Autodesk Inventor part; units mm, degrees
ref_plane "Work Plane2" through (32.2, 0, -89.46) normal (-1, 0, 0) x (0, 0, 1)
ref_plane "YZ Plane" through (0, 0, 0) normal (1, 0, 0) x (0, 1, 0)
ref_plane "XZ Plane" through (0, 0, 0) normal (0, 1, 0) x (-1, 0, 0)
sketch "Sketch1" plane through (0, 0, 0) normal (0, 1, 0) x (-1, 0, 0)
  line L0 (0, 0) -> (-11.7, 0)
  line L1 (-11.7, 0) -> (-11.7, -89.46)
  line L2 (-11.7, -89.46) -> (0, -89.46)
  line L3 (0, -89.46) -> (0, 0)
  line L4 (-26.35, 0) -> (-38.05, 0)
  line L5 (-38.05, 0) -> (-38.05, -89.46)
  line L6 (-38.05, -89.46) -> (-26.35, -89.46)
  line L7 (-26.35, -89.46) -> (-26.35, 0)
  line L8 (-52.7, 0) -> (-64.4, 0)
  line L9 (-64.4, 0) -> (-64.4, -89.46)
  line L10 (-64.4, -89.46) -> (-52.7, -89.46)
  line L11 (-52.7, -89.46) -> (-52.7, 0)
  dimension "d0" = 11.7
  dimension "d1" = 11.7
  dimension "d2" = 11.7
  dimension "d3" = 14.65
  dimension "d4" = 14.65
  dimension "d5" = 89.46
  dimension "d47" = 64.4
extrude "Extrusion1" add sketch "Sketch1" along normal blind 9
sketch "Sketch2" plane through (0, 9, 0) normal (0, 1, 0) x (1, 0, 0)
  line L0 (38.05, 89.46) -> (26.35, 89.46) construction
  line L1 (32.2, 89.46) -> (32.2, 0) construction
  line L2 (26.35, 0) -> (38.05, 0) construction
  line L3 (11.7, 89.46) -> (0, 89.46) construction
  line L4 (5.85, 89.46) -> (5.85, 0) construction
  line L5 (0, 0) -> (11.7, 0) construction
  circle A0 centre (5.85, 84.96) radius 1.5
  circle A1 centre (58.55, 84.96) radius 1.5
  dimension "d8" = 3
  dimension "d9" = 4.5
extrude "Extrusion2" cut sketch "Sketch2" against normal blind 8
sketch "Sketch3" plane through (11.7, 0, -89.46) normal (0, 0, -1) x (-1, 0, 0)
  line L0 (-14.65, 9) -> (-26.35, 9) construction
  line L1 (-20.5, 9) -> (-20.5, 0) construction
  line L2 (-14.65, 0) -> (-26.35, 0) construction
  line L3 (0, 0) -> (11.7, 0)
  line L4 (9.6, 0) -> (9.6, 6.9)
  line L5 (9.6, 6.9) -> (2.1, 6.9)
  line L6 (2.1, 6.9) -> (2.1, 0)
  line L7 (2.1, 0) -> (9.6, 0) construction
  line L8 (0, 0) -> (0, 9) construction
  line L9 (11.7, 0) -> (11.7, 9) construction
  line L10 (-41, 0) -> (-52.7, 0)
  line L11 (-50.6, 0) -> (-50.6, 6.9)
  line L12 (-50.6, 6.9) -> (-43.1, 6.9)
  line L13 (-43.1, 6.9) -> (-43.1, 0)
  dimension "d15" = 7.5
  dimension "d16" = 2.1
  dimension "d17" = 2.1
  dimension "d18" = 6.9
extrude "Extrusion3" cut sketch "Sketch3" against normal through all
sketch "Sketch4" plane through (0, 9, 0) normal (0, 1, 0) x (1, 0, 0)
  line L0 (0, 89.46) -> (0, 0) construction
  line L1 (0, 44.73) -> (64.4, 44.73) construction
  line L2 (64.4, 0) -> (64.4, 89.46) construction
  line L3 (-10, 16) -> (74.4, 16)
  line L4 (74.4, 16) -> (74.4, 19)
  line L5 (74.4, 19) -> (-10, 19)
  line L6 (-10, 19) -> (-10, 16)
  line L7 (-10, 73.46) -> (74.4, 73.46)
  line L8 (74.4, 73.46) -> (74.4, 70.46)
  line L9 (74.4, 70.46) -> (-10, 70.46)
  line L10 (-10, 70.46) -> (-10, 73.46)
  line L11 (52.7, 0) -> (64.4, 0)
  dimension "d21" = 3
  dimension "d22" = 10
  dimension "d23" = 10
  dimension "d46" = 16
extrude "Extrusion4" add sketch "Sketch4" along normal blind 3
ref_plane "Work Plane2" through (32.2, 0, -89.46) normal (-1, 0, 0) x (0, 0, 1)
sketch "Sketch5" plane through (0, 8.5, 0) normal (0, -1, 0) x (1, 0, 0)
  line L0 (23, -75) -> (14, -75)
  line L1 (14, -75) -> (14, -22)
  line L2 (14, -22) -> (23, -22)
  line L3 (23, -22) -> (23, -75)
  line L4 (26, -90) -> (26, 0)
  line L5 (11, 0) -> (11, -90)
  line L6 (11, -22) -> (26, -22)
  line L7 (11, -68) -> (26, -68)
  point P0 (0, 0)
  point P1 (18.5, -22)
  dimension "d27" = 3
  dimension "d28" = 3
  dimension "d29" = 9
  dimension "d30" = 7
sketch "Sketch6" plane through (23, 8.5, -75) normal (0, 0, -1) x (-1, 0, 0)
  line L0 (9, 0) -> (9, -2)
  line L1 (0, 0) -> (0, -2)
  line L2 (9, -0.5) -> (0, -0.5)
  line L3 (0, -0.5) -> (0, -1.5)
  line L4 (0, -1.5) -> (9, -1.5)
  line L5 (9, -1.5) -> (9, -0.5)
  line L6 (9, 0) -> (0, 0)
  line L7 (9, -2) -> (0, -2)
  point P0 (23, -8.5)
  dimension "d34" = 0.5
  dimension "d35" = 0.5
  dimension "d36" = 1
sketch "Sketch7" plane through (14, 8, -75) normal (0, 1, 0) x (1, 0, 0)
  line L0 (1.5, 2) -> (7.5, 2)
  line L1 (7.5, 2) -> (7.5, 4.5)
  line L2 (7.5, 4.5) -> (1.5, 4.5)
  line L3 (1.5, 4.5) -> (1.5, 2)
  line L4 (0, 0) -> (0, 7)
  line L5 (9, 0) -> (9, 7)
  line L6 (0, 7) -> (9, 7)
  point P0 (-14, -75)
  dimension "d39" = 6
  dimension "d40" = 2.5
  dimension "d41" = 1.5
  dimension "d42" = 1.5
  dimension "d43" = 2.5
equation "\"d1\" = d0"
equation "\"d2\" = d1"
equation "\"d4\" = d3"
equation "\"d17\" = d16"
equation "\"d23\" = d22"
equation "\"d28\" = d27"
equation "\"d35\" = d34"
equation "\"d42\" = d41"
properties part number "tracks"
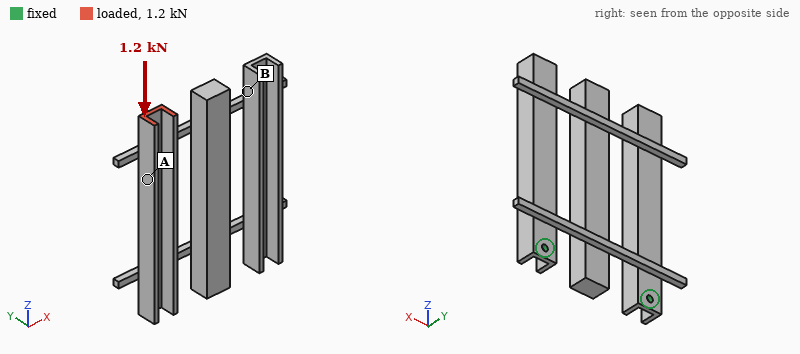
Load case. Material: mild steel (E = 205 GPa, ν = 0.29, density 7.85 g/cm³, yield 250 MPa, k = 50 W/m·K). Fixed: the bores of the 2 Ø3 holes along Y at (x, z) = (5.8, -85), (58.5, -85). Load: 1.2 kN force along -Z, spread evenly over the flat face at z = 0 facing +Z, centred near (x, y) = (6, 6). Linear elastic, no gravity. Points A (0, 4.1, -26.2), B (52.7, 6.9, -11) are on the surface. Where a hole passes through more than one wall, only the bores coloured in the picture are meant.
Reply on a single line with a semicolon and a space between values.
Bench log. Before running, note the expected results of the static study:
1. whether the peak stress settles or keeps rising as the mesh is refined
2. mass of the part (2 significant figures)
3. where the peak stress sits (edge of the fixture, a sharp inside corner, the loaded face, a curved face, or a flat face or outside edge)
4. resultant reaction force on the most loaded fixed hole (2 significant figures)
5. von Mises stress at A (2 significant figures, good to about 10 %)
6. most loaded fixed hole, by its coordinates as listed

keeps rising; 160 g; edge of the fixture; 1.2 kN; 23 MPa; (5.8, -85)
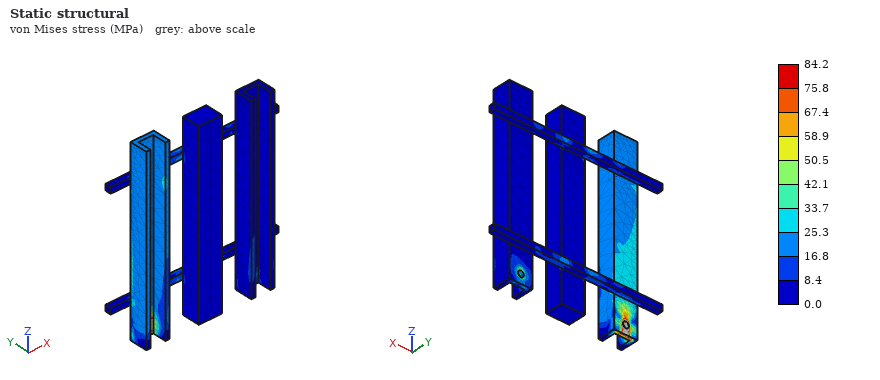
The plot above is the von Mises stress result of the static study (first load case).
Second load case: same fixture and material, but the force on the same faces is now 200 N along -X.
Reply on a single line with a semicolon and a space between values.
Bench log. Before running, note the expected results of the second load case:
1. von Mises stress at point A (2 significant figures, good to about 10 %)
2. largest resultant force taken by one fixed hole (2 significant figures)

31 MPa; 210 N
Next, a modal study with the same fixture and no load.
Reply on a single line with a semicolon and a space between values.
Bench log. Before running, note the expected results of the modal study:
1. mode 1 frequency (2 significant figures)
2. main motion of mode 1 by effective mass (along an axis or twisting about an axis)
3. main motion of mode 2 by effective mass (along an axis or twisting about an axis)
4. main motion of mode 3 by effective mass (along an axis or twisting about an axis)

380 Hz; along Y; along X; along X
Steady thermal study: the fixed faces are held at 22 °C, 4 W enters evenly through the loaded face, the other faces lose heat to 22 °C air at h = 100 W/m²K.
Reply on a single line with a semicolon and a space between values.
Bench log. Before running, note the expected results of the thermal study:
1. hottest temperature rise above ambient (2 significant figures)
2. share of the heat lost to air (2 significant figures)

31 K; 97 %
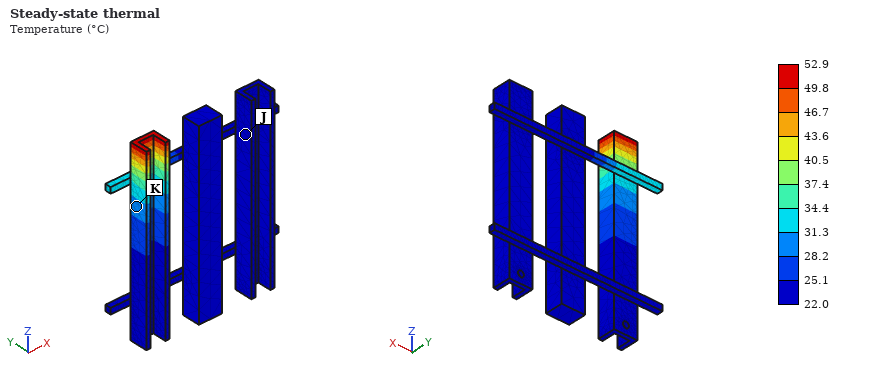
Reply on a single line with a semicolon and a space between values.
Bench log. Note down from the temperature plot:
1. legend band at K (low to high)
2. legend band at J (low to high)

28.2 to 31.3 °C; 22.0 to 25.1 °C
